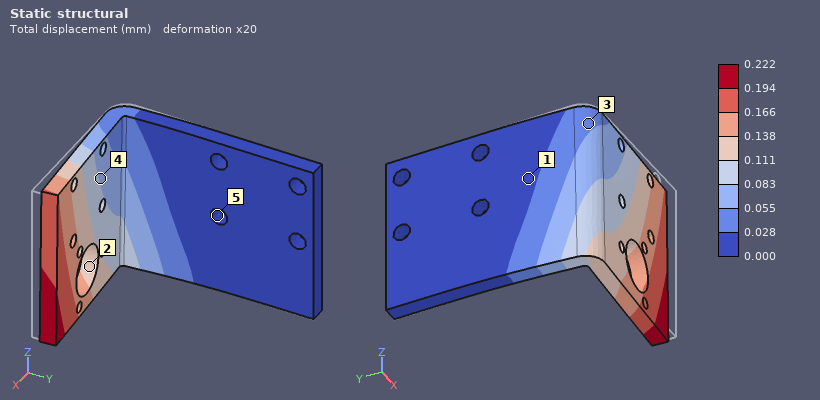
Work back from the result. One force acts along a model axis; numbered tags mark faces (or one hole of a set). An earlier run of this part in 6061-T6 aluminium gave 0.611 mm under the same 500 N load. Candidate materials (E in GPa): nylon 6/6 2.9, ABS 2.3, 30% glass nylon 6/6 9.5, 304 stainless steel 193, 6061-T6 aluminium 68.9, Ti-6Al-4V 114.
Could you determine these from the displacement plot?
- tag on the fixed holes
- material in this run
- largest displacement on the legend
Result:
5
304 stainless steel
0.222 mm
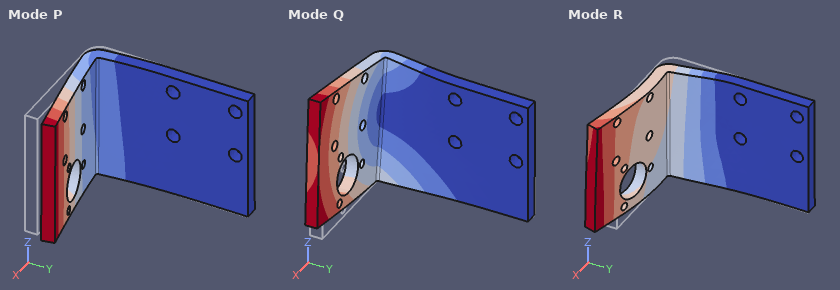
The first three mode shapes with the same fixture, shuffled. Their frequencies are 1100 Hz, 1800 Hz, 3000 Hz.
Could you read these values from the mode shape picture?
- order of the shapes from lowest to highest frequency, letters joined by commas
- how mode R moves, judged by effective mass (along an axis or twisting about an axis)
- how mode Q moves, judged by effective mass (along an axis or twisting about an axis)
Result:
P, Q, R
along X
along Z
